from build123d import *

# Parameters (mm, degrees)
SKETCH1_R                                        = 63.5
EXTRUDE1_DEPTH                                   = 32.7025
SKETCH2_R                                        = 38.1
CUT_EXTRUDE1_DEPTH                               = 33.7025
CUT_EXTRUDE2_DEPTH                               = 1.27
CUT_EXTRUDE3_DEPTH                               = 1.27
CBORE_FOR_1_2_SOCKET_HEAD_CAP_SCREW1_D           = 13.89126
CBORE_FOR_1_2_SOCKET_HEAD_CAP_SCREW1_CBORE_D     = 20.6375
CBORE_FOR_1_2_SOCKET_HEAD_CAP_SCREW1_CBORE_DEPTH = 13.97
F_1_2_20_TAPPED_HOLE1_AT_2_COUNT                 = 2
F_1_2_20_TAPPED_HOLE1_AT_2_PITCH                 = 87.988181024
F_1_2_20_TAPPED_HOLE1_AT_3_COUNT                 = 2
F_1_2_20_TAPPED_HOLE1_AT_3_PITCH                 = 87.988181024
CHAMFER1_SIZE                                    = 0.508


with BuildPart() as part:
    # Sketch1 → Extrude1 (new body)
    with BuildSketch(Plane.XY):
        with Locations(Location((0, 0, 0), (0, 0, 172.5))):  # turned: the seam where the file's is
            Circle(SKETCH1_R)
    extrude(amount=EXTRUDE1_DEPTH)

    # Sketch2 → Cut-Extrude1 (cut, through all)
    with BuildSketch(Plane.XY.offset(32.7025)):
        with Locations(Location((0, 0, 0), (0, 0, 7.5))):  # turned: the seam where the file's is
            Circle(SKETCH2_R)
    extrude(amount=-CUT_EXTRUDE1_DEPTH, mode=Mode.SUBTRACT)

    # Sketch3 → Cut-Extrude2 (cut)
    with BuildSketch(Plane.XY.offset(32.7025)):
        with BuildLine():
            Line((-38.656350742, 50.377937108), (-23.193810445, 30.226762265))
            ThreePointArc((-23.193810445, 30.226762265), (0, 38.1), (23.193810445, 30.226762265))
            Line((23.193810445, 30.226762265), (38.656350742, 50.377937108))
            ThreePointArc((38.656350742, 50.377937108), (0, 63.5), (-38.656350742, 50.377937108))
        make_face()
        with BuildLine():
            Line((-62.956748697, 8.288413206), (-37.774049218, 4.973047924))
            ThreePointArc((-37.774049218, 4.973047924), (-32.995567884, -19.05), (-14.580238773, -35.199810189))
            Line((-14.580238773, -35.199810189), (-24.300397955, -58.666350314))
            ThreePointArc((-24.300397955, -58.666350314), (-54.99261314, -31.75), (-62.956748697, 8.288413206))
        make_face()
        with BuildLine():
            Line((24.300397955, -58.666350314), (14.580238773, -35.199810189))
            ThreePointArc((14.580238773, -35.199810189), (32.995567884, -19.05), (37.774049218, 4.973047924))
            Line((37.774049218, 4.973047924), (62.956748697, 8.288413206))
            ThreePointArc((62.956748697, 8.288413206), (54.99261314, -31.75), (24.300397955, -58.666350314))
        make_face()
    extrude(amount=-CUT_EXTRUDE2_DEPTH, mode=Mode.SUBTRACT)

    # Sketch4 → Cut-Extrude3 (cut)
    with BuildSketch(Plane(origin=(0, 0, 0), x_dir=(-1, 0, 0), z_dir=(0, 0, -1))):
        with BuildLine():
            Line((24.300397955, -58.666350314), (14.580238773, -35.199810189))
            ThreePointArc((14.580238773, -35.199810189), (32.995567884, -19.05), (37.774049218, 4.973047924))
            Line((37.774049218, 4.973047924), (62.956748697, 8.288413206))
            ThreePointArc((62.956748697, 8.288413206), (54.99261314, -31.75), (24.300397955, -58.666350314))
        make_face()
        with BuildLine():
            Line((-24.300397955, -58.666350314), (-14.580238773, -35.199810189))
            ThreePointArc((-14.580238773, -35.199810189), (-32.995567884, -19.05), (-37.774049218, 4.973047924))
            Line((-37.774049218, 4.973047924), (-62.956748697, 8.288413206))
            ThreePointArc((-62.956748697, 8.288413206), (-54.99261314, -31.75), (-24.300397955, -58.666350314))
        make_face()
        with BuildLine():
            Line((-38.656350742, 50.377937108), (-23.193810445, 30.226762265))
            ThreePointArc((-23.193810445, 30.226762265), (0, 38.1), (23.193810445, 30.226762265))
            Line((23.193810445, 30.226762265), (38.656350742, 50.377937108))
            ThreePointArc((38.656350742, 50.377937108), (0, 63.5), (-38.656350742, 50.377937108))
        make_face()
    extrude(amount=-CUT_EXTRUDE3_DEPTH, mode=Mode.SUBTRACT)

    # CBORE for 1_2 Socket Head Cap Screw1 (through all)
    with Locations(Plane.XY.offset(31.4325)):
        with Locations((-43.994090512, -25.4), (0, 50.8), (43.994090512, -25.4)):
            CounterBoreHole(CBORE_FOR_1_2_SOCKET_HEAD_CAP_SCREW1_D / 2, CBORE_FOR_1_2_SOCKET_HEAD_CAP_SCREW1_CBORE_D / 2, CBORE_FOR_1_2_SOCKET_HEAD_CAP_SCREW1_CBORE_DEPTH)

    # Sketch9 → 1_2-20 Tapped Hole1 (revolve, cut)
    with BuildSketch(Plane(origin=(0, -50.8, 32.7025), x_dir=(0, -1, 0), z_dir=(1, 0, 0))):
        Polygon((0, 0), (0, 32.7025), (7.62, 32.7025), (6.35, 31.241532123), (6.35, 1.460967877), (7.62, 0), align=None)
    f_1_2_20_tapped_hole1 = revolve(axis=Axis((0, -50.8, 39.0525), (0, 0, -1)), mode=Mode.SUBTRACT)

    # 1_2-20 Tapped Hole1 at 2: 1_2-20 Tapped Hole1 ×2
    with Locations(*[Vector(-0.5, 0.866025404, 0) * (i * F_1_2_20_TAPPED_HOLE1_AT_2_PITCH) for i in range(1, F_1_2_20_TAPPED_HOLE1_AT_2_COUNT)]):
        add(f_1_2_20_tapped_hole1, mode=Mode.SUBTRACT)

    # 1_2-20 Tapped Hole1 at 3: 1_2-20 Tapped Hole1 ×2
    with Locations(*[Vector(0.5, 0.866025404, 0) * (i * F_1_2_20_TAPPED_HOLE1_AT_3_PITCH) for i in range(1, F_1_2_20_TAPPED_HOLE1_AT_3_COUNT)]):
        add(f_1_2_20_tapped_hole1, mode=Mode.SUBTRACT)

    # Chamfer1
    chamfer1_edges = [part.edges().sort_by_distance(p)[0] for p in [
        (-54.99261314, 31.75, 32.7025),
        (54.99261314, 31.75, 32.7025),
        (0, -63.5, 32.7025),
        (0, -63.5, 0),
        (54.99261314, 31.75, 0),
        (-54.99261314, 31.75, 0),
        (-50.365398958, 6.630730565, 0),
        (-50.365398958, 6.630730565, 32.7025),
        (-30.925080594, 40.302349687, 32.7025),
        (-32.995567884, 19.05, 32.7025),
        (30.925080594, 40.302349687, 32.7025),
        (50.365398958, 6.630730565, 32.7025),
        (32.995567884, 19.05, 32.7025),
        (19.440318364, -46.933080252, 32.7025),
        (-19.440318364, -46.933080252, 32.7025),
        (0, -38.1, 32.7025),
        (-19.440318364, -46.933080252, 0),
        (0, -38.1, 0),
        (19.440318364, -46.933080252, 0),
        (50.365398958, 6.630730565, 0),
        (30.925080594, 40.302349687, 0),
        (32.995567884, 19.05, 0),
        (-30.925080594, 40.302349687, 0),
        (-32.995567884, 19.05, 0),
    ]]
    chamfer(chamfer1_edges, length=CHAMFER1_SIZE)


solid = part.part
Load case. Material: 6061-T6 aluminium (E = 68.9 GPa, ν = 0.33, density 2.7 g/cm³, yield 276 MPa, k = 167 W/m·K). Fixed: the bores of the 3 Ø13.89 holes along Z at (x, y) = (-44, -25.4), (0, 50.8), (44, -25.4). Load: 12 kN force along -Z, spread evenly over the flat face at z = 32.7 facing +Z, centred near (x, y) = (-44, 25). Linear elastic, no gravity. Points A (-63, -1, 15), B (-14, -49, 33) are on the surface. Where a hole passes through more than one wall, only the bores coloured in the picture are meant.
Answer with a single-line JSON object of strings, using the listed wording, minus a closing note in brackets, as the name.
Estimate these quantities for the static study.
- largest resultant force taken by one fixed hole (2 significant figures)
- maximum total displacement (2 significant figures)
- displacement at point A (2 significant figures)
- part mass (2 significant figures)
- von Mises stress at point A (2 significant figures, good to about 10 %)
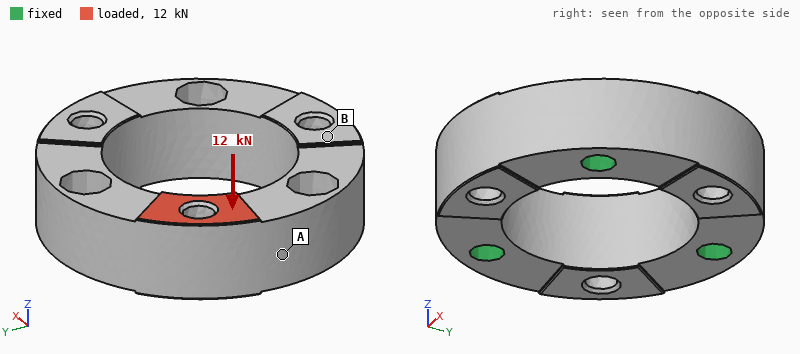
{"largest resultant force taken by one fixed hole": "6.5 kN", "maximum total displacement": "87 µm", "displacement at point A": "41 µm", "part mass": "590 g", "von Mises stress at point A": "31 MPa"}
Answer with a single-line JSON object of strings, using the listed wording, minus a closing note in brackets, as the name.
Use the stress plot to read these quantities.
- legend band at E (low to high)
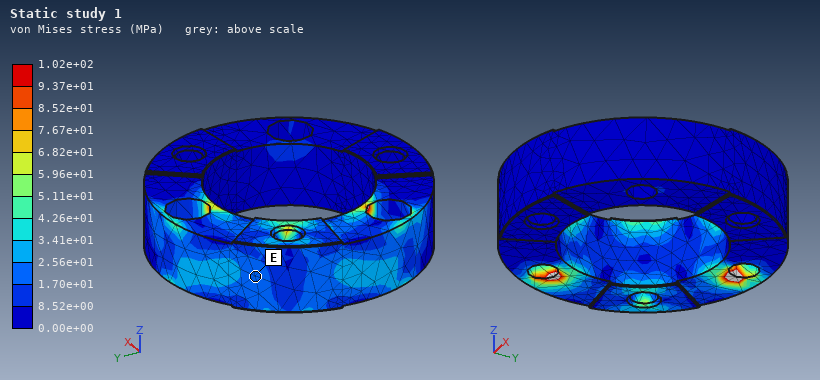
{"legend band at E": "1.70e+01 to 2.56e+01 MPa"}
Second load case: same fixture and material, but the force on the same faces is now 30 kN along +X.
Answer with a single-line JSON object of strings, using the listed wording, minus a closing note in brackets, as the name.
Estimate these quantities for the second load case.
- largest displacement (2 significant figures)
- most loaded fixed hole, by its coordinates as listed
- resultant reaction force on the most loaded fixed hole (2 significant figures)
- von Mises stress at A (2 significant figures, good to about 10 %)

{"largest displacement": "0.22 mm", "most loaded fixed hole, by its coordinates as listed": "(0, 50.8)", "resultant reaction force on the most loaded fixed hole": "23 kN", "von Mises stress at A": "80 MPa"}
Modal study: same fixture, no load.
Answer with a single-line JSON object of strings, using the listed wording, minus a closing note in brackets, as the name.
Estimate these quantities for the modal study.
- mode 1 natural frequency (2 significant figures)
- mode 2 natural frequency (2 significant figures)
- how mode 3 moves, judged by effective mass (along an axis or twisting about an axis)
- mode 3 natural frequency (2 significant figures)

{"mode 1 natural frequency": "6300 Hz", "mode 2 natural frequency": "6300 Hz", "how mode 3 moves, judged by effective mass": "along Z", "mode 3 natural frequency": "7700 Hz"}
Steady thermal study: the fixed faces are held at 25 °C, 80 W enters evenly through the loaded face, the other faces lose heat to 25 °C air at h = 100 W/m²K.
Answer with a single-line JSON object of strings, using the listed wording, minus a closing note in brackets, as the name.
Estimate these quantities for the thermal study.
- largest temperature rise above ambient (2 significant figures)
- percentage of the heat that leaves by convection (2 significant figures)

{"largest temperature rise above ambient": "18 K", "percentage of the heat that leaves by convection": "13 %"}
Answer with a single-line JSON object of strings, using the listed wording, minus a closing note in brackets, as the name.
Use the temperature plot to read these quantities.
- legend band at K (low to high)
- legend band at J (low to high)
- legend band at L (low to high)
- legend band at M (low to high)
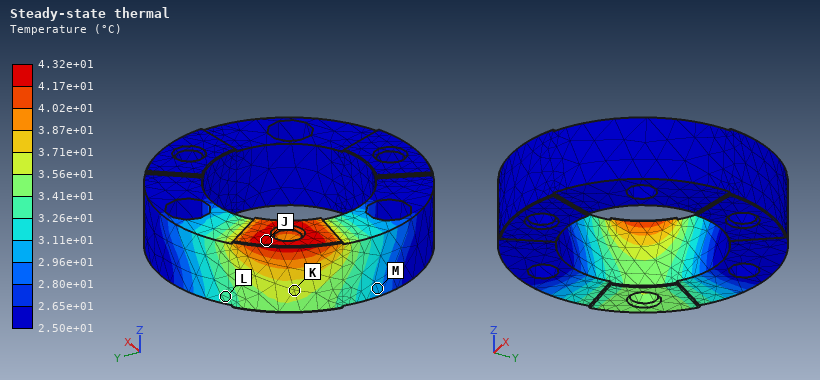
{"legend band at K": "3.56e+01 to 3.71e+01 °C", "legend band at J": "4.17e+01 to 4.32e+01 °C", "legend band at L": "3.26e+01 to 3.41e+01 °C", "legend band at M": "2.96e+01 to 3.11e+01 °C"}
